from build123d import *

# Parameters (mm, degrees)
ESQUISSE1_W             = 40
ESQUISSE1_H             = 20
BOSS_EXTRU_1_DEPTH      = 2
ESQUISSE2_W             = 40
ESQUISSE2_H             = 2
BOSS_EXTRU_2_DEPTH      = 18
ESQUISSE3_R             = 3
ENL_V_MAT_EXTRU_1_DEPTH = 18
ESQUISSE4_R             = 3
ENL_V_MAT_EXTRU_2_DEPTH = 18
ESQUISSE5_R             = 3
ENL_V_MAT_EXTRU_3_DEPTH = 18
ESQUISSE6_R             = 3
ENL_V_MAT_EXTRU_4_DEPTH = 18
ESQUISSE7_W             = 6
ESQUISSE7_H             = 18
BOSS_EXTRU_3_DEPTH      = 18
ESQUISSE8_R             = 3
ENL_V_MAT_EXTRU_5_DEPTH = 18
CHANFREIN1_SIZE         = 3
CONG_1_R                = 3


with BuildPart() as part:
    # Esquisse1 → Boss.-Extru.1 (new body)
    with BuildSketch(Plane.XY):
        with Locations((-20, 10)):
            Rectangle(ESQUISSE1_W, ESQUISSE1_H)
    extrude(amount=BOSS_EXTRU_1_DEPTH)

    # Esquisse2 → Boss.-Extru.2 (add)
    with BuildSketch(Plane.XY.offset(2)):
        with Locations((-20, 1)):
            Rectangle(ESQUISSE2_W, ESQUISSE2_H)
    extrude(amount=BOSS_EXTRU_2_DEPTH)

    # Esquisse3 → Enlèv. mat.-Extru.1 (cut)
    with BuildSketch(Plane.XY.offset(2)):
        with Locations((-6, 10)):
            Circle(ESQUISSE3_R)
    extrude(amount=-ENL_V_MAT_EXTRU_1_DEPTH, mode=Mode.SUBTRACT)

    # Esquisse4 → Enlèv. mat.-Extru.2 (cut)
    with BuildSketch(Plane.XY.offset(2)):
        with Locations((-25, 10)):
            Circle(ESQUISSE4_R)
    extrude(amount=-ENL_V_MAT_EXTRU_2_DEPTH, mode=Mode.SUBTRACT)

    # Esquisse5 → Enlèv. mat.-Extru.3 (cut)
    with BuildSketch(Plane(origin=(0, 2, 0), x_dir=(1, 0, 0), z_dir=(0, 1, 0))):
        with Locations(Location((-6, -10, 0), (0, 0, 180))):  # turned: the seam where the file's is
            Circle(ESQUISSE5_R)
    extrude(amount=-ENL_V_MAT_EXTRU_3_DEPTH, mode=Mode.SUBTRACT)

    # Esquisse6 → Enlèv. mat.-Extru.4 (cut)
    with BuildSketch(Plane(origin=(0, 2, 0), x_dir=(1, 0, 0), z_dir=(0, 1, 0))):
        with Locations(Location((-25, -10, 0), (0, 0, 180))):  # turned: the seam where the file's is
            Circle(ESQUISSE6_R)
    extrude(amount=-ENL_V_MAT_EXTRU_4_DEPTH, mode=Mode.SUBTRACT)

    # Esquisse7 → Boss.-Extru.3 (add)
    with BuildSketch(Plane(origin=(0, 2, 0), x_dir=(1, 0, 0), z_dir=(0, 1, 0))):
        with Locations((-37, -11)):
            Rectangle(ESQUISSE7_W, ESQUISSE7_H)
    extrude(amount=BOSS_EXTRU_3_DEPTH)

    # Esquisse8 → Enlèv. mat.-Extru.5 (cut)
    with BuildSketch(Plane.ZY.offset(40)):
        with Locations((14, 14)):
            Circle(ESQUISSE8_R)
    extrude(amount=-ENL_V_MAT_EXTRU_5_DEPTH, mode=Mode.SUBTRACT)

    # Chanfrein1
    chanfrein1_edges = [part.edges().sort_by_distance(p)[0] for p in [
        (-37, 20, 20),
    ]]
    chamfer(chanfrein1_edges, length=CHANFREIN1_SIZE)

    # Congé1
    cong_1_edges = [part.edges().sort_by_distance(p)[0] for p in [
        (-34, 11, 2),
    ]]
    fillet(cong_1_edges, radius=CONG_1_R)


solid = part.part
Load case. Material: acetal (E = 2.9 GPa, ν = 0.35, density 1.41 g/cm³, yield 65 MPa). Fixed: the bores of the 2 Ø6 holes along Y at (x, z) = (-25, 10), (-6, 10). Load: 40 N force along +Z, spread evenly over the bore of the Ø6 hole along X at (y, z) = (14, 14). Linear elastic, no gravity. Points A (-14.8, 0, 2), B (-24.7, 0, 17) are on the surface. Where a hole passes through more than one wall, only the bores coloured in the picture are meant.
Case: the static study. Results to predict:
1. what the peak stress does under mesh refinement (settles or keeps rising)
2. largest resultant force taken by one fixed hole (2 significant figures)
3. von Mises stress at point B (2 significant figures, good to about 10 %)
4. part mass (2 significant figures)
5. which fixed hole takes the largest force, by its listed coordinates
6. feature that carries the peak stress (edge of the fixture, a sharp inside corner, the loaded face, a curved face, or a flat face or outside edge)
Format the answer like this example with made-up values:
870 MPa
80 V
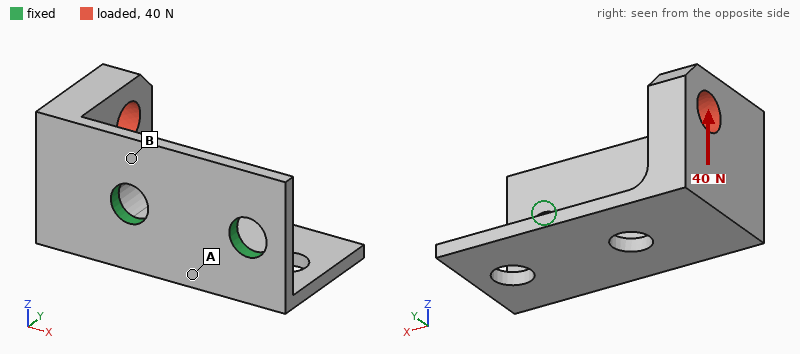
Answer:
keeps rising
52 N
11 MPa
6.5 g
(-25, 10)
edge of the fixture
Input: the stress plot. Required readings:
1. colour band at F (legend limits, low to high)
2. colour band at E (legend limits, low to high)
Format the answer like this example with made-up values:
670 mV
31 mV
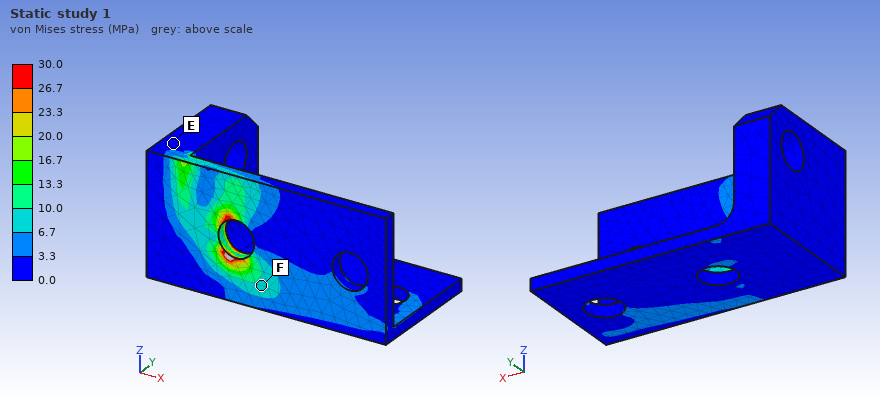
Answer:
6.7 to 10.0 MPa
0.0 to 3.3 MPa
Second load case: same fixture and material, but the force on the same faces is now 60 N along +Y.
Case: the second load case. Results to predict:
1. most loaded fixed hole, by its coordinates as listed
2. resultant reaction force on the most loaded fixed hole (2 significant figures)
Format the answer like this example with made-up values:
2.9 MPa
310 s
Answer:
(-25, 10)
78 N
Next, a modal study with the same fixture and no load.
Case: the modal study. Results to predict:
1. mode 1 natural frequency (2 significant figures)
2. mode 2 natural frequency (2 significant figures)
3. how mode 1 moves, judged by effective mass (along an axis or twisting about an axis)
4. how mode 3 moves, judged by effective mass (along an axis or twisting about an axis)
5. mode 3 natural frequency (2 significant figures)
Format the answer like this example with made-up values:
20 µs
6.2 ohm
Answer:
890 Hz
1200 Hz
along Z
along Y
1700 Hz
